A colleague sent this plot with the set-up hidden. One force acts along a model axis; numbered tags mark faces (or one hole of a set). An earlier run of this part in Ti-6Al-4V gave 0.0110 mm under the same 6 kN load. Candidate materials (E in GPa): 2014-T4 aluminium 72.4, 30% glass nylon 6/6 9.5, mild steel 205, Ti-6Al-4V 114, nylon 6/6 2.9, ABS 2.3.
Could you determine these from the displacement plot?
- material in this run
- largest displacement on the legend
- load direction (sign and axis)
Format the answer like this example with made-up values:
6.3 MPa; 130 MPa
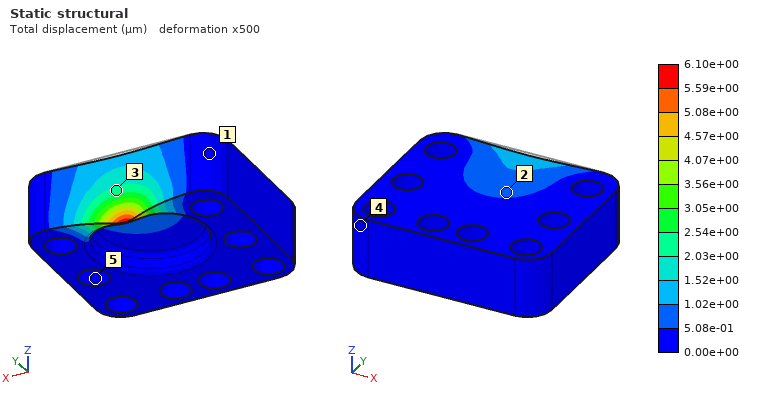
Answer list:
mild steel; 6.10e+00 µm; -Y
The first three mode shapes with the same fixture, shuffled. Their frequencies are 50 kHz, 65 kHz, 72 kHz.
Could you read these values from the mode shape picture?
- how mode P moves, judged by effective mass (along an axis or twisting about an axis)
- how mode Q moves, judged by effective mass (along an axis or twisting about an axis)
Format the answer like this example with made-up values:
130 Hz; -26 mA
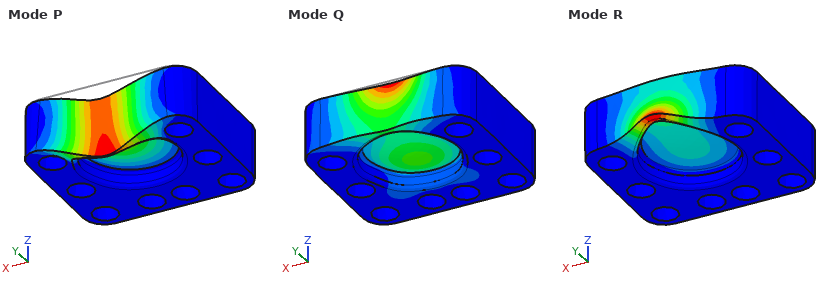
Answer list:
along Z; along Y
